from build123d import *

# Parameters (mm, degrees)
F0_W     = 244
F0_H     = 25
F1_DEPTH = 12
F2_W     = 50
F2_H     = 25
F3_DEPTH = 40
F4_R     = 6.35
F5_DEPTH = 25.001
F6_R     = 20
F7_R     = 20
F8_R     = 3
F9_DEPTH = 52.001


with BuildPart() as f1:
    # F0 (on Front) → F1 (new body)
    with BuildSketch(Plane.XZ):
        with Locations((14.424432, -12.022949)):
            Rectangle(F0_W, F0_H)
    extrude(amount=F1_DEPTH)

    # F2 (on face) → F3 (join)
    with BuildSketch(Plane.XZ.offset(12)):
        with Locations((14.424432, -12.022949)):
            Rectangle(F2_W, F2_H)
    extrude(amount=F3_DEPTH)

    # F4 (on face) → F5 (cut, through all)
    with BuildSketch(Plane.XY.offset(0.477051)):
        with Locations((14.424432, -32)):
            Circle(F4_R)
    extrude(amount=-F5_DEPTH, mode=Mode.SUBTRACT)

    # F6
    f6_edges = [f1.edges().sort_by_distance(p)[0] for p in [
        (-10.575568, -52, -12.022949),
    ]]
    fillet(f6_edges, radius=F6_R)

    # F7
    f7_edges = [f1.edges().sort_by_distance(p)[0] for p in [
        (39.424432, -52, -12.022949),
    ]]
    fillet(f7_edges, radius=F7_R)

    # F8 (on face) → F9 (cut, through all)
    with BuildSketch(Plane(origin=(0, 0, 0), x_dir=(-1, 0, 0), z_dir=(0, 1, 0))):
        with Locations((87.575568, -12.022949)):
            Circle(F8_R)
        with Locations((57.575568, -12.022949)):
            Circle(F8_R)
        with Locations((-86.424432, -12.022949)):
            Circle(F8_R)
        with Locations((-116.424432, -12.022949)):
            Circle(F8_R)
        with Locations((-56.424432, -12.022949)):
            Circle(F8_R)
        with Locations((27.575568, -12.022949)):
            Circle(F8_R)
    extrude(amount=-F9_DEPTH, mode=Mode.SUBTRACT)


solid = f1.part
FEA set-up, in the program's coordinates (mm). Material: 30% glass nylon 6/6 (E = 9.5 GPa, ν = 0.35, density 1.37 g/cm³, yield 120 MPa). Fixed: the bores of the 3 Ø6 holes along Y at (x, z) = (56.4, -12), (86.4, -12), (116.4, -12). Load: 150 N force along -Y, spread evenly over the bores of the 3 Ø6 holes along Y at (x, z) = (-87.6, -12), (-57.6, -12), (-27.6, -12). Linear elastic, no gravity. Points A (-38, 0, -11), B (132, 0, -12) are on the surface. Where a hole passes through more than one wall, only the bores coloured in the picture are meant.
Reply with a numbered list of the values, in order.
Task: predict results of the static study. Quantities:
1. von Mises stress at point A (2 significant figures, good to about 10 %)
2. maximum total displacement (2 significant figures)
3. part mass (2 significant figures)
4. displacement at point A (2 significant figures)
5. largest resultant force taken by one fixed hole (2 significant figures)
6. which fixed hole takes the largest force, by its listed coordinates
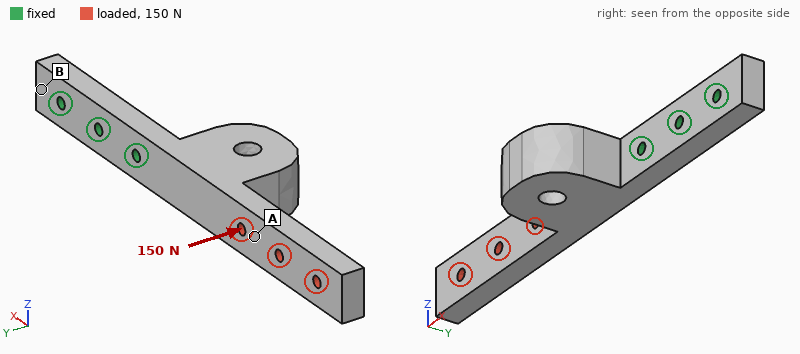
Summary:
1. 5.2 MPa
2. 2.3 mm
3. 160 g
4. 1.0 mm
5. 290 N
6. (56.4, -12)
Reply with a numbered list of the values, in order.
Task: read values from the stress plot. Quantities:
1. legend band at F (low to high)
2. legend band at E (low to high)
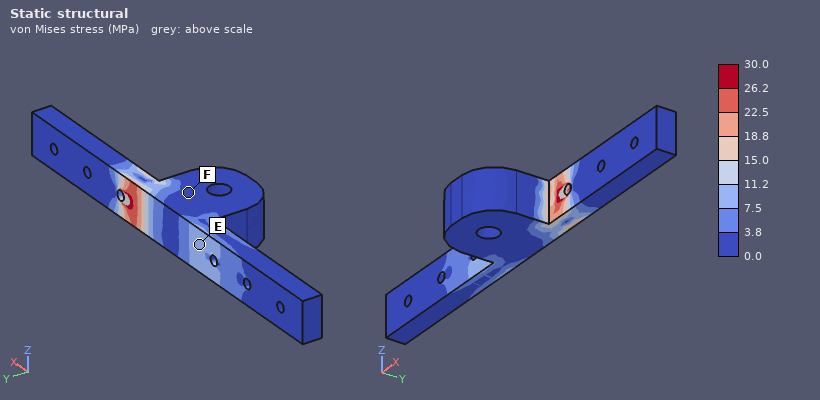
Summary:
1. 0.0 to 3.8 MPa
2. 7.5 to 11.2 MPa
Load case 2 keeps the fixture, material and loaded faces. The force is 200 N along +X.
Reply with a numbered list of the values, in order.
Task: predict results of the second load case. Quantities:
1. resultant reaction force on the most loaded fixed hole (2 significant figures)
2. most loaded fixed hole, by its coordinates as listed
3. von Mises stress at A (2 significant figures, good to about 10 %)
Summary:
1. 170 N
2. (56.4, -12)
3. 0.28 MPa
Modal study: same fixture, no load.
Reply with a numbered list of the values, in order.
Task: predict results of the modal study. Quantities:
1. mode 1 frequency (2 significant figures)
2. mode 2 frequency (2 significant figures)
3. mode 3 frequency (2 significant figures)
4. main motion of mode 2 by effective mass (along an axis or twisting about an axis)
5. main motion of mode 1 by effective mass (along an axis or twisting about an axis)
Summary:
1. 230 Hz
2. 370 Hz
3. 860 Hz
4. along Z
5. along Y
